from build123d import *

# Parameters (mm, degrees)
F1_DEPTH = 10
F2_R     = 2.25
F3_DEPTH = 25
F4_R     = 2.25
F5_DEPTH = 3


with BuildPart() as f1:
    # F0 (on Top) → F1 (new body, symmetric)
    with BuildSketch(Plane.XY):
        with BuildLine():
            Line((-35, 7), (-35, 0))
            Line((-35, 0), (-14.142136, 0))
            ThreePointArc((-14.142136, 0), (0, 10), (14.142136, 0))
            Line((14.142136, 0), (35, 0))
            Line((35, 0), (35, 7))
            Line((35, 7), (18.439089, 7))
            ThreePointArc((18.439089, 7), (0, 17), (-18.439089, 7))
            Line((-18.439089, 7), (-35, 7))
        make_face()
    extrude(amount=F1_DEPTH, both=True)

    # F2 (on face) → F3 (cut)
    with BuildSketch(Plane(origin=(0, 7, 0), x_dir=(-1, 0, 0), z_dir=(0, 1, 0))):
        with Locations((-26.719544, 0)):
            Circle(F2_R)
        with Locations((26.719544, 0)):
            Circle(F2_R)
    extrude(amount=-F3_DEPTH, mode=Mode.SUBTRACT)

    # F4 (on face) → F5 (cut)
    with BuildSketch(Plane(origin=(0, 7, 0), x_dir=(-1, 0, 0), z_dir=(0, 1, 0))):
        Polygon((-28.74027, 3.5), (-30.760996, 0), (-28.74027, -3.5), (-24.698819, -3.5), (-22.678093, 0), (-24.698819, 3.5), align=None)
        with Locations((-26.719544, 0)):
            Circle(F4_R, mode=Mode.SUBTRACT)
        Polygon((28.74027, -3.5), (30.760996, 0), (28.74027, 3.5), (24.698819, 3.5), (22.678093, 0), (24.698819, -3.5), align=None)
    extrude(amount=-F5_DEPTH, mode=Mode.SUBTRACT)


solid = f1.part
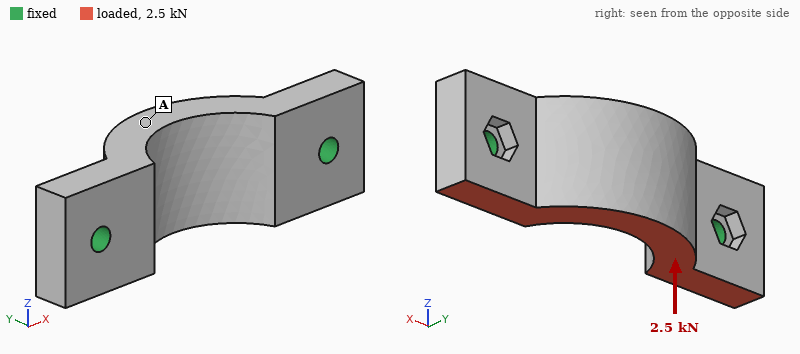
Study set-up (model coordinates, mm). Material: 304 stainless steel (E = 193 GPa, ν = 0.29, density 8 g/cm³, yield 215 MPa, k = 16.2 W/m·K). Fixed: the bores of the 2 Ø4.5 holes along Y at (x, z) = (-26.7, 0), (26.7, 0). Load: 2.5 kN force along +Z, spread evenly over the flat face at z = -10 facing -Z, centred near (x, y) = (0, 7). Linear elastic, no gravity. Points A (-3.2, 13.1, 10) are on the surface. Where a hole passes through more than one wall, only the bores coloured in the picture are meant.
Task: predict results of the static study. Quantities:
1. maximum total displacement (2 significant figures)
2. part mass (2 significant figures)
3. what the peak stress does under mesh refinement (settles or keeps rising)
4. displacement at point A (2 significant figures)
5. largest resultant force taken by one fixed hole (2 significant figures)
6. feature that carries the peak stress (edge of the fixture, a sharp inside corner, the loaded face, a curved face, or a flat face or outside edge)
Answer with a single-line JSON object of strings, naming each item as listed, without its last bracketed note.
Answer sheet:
{"maximum total displacement": "21 µm", "part mass": "84 g", "what the peak stress does under mesh refinement": "keeps rising", "displacement at point A": "17 µm", "largest resultant force taken by one fixed hole": "1.3 kN", "feature that carries the peak stress": "edge of the fixture"}
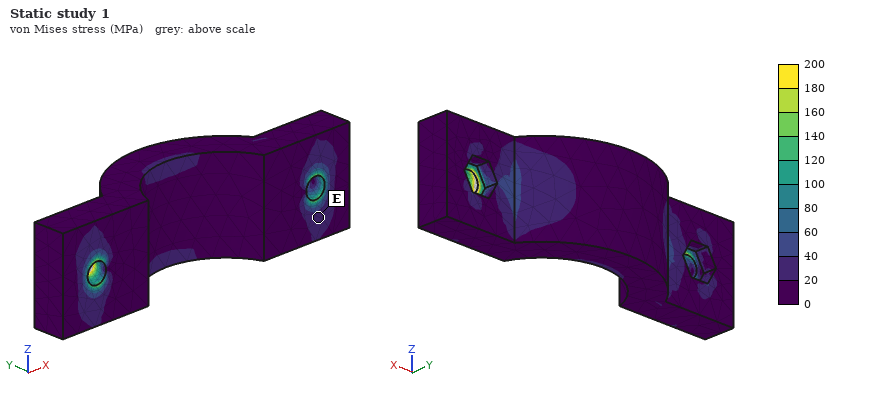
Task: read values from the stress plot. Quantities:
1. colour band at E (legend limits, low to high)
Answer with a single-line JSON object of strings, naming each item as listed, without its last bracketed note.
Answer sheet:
{"colour band at E": "20 to 40 MPa"}
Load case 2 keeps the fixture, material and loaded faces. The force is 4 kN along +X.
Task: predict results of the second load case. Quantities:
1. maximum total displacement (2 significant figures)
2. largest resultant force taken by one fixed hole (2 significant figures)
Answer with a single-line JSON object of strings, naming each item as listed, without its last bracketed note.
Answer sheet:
{"maximum total displacement": "6.3 µm", "largest resultant force taken by one fixed hole": "2.1 kN"}
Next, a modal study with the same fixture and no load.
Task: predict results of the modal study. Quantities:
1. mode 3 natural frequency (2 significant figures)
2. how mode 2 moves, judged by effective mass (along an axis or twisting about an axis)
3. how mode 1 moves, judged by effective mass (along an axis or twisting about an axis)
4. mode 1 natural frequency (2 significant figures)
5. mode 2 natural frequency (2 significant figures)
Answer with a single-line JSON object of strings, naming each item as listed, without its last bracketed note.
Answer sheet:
{"mode 3 natural frequency": "19 kHz", "how mode 2 moves, judged by effective mass": "along Y", "how mode 1 moves, judged by effective mass": "along Z", "mode 1 natural frequency": "7000 Hz", "mode 2 natural frequency": "14 kHz"}
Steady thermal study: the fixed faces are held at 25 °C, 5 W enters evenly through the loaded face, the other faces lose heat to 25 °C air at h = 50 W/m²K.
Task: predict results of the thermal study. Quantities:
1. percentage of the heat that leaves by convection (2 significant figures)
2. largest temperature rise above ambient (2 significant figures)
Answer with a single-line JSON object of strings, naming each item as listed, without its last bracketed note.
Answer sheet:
{"percentage of the heat that leaves by convection": "28 %", "largest temperature rise above ambient": "15 K"}
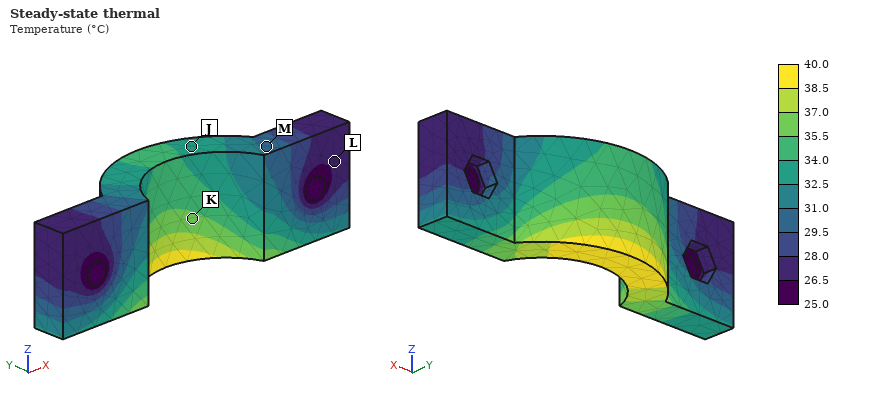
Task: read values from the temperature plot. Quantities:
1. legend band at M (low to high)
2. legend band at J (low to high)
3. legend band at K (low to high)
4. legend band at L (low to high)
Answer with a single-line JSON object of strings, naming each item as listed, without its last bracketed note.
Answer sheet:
{"legend band at M": "29.5 to 31.0 °C", "legend band at J": "32.5 to 34.0 °C", "legend band at K": "35.5 to 37.0 °C", "legend band at L": "26.5 to 28.0 °C"}
